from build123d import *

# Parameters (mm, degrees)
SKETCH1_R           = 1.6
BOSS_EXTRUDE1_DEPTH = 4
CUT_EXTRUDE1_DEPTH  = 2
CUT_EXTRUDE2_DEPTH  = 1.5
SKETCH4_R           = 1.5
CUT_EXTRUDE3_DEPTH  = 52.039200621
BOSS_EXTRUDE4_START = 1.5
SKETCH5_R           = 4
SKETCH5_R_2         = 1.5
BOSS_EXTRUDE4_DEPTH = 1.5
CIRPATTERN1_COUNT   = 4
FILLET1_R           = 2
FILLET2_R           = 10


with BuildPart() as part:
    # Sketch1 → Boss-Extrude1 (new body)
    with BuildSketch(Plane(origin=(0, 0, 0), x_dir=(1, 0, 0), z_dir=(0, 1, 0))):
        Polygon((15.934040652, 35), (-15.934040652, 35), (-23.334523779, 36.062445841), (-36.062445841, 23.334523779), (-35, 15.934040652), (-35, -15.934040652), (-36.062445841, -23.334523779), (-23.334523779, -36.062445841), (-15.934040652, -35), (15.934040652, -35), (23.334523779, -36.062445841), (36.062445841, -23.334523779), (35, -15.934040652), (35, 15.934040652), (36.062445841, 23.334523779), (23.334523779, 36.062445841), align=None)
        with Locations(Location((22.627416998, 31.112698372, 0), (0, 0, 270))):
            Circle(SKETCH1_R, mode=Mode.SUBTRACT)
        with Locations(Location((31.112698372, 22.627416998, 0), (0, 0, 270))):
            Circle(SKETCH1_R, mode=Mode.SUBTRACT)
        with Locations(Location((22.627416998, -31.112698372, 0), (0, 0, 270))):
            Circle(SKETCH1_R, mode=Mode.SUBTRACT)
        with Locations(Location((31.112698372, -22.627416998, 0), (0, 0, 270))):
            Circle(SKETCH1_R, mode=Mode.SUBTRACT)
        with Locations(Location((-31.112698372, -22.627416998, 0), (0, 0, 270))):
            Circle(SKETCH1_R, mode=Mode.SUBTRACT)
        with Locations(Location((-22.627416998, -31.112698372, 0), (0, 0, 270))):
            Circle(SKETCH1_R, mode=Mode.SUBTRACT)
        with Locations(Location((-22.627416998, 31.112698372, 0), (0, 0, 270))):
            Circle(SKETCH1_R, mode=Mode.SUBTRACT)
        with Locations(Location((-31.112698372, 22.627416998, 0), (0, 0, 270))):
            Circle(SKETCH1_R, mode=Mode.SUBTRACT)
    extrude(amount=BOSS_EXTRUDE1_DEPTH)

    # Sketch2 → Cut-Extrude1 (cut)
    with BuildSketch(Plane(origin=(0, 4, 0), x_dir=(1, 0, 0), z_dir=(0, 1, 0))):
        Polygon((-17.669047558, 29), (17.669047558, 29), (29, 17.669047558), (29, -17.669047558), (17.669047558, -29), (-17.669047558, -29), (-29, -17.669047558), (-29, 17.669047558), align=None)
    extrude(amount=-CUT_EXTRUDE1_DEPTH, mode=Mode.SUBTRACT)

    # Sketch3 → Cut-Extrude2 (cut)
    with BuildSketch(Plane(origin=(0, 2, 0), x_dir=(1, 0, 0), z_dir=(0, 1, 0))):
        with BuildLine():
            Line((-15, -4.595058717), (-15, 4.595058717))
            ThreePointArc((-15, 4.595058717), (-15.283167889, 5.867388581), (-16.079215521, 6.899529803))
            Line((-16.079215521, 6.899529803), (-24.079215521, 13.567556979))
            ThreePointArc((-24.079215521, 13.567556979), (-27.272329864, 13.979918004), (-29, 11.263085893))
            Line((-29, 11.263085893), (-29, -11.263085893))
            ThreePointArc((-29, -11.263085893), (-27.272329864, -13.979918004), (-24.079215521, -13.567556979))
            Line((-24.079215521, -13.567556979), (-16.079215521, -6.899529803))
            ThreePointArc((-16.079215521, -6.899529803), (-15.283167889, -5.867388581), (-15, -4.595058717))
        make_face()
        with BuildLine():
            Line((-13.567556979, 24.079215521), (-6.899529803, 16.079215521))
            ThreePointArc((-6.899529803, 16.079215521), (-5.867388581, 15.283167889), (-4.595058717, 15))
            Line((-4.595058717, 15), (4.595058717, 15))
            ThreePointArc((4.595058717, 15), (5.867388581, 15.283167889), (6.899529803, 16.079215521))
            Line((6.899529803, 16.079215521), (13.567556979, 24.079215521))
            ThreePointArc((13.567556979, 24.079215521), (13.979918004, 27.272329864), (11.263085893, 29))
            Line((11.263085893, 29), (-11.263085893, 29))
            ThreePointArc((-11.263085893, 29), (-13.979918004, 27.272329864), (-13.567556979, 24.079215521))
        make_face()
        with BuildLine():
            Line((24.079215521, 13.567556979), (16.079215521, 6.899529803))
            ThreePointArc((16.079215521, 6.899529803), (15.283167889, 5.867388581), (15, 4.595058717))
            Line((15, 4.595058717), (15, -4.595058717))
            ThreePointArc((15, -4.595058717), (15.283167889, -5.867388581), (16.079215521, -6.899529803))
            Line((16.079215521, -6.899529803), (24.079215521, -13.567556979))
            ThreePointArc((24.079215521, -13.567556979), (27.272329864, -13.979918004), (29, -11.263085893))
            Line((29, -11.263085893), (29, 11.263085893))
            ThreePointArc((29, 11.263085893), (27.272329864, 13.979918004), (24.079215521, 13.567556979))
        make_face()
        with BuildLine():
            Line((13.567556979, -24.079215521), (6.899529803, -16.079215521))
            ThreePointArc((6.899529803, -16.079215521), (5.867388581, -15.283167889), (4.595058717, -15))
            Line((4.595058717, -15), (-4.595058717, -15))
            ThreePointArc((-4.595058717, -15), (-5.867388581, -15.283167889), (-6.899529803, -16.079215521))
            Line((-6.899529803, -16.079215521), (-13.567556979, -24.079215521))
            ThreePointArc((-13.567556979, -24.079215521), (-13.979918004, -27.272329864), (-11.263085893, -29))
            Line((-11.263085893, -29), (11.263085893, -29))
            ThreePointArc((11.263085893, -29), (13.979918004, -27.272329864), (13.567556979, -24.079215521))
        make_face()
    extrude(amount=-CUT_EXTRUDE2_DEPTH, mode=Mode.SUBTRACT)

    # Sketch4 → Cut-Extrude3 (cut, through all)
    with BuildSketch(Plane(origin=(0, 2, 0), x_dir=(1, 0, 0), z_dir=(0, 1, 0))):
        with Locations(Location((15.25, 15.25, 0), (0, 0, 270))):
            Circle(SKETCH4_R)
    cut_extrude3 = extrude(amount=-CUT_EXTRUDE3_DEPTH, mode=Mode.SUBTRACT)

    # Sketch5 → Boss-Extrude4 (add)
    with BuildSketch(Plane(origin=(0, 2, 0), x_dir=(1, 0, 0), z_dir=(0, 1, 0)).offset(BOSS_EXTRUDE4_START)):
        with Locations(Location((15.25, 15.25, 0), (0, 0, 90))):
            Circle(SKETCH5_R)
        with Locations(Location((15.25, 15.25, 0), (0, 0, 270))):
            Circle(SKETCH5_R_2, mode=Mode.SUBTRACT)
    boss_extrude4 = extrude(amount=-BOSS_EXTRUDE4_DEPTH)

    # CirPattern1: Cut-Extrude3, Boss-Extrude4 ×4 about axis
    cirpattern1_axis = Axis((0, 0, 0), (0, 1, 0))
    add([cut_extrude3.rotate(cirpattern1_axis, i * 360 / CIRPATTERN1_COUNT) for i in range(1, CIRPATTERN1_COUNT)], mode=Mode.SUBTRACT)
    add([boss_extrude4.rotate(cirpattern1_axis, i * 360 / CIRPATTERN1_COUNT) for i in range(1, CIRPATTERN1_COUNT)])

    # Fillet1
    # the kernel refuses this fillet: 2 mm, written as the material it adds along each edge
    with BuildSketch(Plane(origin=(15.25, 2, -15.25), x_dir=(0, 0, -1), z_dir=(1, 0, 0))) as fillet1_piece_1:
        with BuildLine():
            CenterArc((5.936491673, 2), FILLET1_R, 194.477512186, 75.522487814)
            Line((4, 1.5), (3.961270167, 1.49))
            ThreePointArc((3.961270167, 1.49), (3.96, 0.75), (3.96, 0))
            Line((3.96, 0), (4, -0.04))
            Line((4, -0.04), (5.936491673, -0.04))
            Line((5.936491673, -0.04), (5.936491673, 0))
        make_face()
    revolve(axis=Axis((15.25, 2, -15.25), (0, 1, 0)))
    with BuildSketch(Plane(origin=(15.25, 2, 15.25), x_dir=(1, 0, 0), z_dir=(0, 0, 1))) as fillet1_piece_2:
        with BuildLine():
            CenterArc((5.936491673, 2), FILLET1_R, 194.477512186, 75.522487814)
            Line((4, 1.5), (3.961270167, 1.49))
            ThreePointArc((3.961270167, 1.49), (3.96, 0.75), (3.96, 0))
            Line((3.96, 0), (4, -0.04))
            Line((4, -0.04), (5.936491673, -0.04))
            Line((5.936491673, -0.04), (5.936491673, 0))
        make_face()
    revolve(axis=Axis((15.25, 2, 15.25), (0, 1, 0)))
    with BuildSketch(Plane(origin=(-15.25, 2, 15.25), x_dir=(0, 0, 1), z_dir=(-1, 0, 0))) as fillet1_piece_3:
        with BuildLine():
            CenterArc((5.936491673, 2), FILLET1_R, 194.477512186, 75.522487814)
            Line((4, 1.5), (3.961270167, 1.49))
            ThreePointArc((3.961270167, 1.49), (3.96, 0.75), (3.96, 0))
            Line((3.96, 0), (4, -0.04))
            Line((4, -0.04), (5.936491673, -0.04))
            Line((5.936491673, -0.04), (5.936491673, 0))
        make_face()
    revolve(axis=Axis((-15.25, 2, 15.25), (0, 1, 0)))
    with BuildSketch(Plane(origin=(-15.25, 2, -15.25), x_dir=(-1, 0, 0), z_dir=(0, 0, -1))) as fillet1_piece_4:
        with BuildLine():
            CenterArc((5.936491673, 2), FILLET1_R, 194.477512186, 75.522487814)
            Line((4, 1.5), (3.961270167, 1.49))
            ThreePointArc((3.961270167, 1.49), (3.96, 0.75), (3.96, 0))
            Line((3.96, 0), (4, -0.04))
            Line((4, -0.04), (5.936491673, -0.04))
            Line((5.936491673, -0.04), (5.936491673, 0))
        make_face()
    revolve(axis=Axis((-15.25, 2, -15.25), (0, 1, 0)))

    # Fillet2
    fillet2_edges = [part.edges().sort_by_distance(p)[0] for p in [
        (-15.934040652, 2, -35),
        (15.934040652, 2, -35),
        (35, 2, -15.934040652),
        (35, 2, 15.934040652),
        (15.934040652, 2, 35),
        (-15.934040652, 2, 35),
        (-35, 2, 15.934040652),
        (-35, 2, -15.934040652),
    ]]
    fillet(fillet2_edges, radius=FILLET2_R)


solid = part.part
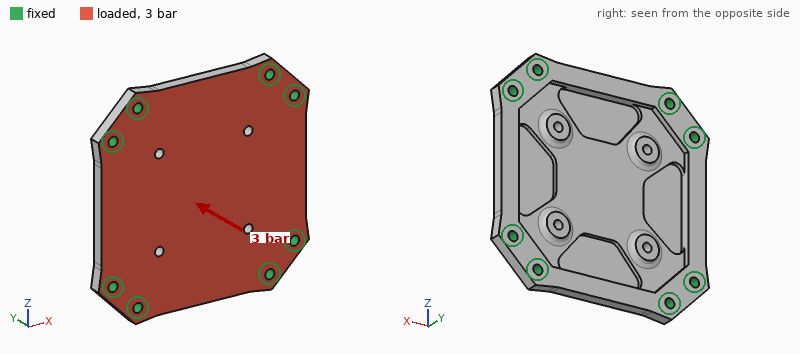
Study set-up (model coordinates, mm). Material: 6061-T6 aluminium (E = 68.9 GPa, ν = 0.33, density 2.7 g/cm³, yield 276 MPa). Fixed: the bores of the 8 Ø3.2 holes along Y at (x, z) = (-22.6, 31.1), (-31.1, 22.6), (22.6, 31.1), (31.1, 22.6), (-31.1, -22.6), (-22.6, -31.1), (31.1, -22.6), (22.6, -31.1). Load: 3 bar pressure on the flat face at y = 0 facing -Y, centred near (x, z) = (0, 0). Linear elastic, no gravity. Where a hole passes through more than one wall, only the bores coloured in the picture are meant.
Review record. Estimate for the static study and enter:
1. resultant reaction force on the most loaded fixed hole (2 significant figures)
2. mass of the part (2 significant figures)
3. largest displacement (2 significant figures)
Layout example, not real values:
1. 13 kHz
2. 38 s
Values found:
1. 210 N
2. 29 g
3. 0.22 mm
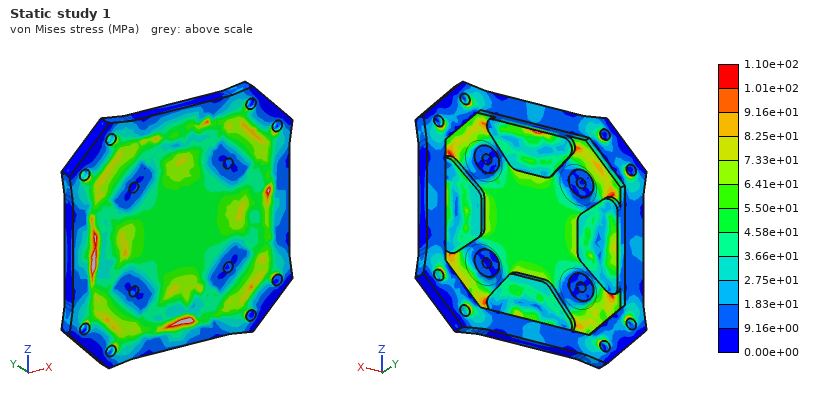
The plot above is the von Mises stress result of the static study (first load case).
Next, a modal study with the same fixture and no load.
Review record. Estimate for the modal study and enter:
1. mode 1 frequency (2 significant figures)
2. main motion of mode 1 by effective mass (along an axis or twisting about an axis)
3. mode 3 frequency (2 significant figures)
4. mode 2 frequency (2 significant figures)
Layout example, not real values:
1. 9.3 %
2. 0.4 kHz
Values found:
1. 3300 Hz
2. along Y
3. 7200 Hz
4. 7200 Hz
